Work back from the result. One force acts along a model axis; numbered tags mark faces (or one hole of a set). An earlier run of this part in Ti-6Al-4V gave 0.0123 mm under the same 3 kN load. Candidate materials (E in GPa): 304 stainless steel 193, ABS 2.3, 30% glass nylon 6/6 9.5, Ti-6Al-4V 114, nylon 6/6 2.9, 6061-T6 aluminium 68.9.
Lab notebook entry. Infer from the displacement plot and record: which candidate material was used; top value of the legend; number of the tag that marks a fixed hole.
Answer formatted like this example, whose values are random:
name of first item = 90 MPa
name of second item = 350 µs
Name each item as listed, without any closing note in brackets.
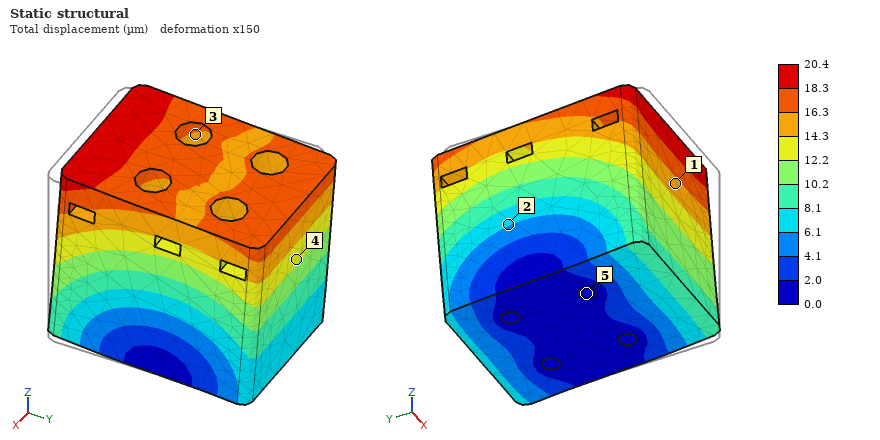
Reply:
which candidate material was used = 6061-T6 aluminium
top value of the legend = 20.4 µm
number of the tag that marks a fixed hole = 5
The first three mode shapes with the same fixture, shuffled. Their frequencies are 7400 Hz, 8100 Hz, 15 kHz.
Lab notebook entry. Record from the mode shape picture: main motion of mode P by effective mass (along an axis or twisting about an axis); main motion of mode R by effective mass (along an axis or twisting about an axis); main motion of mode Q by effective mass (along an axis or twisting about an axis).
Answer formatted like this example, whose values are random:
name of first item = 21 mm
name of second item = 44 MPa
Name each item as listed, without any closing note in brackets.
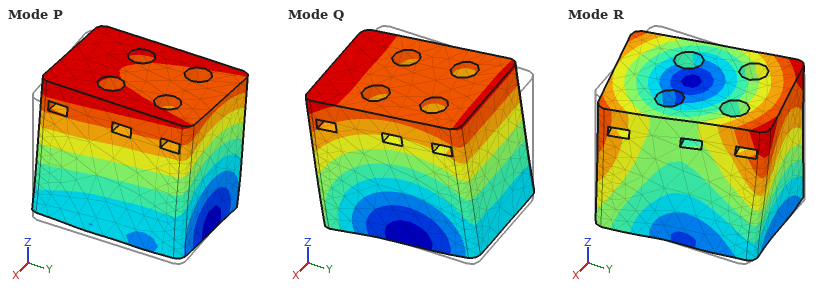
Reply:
main motion of mode P by effective mass = along X
main motion of mode R by effective mass = twisting about Z
main motion of mode Q by effective mass = along Y
